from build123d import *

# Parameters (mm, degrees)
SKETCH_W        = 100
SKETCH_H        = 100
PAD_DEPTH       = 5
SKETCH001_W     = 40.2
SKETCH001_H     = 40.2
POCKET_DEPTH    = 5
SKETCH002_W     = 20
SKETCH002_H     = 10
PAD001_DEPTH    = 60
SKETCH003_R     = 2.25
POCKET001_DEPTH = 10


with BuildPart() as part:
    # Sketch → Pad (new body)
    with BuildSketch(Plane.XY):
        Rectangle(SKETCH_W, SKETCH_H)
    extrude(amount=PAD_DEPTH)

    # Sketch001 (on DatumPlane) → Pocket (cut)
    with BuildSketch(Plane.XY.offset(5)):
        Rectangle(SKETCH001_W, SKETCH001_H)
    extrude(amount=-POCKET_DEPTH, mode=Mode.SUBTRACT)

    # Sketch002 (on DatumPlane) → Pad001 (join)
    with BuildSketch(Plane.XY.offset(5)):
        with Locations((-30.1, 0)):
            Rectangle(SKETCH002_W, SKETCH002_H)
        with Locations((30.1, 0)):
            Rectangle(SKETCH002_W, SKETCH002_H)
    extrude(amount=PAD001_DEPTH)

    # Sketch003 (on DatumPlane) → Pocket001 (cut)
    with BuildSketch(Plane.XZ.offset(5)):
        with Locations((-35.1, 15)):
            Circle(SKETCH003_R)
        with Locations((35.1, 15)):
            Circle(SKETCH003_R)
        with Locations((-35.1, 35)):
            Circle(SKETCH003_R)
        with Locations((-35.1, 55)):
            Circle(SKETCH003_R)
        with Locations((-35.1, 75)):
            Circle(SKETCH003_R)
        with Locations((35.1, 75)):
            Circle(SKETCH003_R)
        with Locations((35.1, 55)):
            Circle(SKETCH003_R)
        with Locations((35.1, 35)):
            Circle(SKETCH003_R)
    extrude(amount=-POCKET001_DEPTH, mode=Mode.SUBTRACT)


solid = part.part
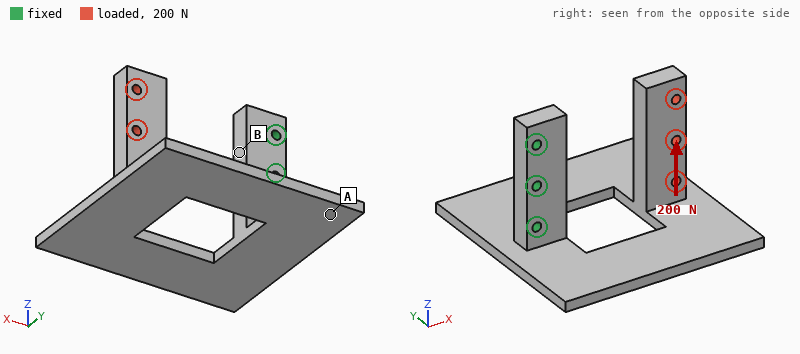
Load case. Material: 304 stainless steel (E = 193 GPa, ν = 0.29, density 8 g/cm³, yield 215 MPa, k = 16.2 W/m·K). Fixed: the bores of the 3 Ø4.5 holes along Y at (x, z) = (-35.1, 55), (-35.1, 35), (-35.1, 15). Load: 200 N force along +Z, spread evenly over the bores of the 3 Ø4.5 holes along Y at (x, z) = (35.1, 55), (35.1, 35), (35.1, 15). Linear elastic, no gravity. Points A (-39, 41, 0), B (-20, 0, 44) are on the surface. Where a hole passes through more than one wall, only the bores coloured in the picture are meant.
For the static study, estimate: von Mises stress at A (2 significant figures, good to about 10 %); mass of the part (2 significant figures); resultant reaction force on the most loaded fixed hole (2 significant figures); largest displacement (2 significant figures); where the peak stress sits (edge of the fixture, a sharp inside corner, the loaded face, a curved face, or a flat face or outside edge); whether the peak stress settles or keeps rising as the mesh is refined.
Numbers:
16 MPa
520 g
550 N
0.44 mm
a sharp inside corner
keeps rising
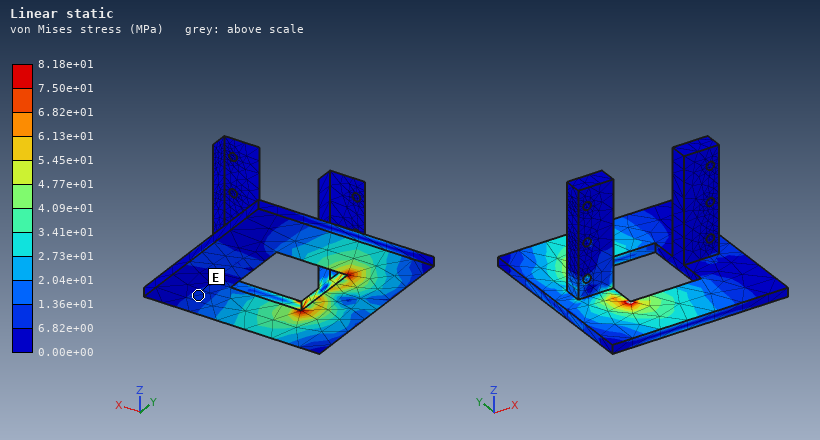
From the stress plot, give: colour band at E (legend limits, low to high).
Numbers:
6.82e+00 to 1.36e+01 MPa
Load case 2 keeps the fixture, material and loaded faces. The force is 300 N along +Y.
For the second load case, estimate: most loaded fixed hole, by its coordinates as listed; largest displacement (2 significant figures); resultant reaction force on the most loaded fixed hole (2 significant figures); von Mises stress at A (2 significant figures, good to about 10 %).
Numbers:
(-35.1, 15)
0.36 mm
200 N
16 MPa
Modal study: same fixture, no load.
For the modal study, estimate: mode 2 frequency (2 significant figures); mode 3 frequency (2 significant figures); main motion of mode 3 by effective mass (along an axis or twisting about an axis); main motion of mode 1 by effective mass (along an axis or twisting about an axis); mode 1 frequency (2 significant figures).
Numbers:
450 Hz
680 Hz
along Y
along Z
270 Hz
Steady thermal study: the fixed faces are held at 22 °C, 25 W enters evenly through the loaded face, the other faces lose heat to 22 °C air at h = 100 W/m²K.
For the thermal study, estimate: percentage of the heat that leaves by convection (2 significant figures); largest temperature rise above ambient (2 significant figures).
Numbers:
100 %
74 K
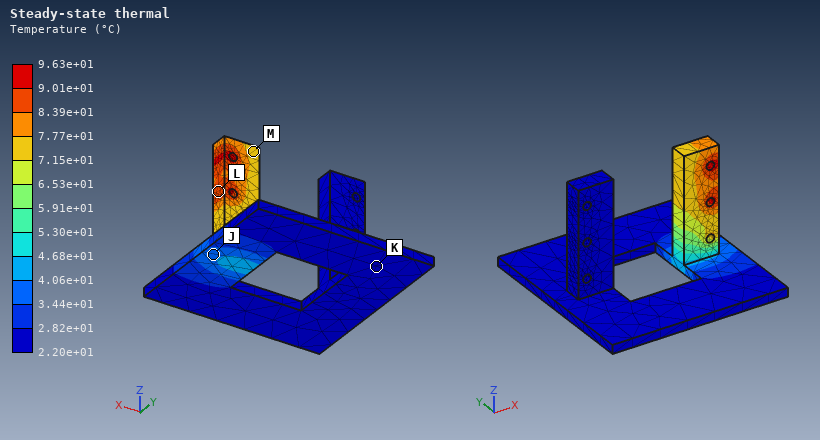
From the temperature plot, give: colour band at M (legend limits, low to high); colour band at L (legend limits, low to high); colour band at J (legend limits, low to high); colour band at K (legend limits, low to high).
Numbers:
7.15e+01 to 7.77e+01 °C
8.39e+01 to 9.01e+01 °C
3.44e+01 to 4.06e+01 °C
2.20e+01 to 2.82e+01 °C
